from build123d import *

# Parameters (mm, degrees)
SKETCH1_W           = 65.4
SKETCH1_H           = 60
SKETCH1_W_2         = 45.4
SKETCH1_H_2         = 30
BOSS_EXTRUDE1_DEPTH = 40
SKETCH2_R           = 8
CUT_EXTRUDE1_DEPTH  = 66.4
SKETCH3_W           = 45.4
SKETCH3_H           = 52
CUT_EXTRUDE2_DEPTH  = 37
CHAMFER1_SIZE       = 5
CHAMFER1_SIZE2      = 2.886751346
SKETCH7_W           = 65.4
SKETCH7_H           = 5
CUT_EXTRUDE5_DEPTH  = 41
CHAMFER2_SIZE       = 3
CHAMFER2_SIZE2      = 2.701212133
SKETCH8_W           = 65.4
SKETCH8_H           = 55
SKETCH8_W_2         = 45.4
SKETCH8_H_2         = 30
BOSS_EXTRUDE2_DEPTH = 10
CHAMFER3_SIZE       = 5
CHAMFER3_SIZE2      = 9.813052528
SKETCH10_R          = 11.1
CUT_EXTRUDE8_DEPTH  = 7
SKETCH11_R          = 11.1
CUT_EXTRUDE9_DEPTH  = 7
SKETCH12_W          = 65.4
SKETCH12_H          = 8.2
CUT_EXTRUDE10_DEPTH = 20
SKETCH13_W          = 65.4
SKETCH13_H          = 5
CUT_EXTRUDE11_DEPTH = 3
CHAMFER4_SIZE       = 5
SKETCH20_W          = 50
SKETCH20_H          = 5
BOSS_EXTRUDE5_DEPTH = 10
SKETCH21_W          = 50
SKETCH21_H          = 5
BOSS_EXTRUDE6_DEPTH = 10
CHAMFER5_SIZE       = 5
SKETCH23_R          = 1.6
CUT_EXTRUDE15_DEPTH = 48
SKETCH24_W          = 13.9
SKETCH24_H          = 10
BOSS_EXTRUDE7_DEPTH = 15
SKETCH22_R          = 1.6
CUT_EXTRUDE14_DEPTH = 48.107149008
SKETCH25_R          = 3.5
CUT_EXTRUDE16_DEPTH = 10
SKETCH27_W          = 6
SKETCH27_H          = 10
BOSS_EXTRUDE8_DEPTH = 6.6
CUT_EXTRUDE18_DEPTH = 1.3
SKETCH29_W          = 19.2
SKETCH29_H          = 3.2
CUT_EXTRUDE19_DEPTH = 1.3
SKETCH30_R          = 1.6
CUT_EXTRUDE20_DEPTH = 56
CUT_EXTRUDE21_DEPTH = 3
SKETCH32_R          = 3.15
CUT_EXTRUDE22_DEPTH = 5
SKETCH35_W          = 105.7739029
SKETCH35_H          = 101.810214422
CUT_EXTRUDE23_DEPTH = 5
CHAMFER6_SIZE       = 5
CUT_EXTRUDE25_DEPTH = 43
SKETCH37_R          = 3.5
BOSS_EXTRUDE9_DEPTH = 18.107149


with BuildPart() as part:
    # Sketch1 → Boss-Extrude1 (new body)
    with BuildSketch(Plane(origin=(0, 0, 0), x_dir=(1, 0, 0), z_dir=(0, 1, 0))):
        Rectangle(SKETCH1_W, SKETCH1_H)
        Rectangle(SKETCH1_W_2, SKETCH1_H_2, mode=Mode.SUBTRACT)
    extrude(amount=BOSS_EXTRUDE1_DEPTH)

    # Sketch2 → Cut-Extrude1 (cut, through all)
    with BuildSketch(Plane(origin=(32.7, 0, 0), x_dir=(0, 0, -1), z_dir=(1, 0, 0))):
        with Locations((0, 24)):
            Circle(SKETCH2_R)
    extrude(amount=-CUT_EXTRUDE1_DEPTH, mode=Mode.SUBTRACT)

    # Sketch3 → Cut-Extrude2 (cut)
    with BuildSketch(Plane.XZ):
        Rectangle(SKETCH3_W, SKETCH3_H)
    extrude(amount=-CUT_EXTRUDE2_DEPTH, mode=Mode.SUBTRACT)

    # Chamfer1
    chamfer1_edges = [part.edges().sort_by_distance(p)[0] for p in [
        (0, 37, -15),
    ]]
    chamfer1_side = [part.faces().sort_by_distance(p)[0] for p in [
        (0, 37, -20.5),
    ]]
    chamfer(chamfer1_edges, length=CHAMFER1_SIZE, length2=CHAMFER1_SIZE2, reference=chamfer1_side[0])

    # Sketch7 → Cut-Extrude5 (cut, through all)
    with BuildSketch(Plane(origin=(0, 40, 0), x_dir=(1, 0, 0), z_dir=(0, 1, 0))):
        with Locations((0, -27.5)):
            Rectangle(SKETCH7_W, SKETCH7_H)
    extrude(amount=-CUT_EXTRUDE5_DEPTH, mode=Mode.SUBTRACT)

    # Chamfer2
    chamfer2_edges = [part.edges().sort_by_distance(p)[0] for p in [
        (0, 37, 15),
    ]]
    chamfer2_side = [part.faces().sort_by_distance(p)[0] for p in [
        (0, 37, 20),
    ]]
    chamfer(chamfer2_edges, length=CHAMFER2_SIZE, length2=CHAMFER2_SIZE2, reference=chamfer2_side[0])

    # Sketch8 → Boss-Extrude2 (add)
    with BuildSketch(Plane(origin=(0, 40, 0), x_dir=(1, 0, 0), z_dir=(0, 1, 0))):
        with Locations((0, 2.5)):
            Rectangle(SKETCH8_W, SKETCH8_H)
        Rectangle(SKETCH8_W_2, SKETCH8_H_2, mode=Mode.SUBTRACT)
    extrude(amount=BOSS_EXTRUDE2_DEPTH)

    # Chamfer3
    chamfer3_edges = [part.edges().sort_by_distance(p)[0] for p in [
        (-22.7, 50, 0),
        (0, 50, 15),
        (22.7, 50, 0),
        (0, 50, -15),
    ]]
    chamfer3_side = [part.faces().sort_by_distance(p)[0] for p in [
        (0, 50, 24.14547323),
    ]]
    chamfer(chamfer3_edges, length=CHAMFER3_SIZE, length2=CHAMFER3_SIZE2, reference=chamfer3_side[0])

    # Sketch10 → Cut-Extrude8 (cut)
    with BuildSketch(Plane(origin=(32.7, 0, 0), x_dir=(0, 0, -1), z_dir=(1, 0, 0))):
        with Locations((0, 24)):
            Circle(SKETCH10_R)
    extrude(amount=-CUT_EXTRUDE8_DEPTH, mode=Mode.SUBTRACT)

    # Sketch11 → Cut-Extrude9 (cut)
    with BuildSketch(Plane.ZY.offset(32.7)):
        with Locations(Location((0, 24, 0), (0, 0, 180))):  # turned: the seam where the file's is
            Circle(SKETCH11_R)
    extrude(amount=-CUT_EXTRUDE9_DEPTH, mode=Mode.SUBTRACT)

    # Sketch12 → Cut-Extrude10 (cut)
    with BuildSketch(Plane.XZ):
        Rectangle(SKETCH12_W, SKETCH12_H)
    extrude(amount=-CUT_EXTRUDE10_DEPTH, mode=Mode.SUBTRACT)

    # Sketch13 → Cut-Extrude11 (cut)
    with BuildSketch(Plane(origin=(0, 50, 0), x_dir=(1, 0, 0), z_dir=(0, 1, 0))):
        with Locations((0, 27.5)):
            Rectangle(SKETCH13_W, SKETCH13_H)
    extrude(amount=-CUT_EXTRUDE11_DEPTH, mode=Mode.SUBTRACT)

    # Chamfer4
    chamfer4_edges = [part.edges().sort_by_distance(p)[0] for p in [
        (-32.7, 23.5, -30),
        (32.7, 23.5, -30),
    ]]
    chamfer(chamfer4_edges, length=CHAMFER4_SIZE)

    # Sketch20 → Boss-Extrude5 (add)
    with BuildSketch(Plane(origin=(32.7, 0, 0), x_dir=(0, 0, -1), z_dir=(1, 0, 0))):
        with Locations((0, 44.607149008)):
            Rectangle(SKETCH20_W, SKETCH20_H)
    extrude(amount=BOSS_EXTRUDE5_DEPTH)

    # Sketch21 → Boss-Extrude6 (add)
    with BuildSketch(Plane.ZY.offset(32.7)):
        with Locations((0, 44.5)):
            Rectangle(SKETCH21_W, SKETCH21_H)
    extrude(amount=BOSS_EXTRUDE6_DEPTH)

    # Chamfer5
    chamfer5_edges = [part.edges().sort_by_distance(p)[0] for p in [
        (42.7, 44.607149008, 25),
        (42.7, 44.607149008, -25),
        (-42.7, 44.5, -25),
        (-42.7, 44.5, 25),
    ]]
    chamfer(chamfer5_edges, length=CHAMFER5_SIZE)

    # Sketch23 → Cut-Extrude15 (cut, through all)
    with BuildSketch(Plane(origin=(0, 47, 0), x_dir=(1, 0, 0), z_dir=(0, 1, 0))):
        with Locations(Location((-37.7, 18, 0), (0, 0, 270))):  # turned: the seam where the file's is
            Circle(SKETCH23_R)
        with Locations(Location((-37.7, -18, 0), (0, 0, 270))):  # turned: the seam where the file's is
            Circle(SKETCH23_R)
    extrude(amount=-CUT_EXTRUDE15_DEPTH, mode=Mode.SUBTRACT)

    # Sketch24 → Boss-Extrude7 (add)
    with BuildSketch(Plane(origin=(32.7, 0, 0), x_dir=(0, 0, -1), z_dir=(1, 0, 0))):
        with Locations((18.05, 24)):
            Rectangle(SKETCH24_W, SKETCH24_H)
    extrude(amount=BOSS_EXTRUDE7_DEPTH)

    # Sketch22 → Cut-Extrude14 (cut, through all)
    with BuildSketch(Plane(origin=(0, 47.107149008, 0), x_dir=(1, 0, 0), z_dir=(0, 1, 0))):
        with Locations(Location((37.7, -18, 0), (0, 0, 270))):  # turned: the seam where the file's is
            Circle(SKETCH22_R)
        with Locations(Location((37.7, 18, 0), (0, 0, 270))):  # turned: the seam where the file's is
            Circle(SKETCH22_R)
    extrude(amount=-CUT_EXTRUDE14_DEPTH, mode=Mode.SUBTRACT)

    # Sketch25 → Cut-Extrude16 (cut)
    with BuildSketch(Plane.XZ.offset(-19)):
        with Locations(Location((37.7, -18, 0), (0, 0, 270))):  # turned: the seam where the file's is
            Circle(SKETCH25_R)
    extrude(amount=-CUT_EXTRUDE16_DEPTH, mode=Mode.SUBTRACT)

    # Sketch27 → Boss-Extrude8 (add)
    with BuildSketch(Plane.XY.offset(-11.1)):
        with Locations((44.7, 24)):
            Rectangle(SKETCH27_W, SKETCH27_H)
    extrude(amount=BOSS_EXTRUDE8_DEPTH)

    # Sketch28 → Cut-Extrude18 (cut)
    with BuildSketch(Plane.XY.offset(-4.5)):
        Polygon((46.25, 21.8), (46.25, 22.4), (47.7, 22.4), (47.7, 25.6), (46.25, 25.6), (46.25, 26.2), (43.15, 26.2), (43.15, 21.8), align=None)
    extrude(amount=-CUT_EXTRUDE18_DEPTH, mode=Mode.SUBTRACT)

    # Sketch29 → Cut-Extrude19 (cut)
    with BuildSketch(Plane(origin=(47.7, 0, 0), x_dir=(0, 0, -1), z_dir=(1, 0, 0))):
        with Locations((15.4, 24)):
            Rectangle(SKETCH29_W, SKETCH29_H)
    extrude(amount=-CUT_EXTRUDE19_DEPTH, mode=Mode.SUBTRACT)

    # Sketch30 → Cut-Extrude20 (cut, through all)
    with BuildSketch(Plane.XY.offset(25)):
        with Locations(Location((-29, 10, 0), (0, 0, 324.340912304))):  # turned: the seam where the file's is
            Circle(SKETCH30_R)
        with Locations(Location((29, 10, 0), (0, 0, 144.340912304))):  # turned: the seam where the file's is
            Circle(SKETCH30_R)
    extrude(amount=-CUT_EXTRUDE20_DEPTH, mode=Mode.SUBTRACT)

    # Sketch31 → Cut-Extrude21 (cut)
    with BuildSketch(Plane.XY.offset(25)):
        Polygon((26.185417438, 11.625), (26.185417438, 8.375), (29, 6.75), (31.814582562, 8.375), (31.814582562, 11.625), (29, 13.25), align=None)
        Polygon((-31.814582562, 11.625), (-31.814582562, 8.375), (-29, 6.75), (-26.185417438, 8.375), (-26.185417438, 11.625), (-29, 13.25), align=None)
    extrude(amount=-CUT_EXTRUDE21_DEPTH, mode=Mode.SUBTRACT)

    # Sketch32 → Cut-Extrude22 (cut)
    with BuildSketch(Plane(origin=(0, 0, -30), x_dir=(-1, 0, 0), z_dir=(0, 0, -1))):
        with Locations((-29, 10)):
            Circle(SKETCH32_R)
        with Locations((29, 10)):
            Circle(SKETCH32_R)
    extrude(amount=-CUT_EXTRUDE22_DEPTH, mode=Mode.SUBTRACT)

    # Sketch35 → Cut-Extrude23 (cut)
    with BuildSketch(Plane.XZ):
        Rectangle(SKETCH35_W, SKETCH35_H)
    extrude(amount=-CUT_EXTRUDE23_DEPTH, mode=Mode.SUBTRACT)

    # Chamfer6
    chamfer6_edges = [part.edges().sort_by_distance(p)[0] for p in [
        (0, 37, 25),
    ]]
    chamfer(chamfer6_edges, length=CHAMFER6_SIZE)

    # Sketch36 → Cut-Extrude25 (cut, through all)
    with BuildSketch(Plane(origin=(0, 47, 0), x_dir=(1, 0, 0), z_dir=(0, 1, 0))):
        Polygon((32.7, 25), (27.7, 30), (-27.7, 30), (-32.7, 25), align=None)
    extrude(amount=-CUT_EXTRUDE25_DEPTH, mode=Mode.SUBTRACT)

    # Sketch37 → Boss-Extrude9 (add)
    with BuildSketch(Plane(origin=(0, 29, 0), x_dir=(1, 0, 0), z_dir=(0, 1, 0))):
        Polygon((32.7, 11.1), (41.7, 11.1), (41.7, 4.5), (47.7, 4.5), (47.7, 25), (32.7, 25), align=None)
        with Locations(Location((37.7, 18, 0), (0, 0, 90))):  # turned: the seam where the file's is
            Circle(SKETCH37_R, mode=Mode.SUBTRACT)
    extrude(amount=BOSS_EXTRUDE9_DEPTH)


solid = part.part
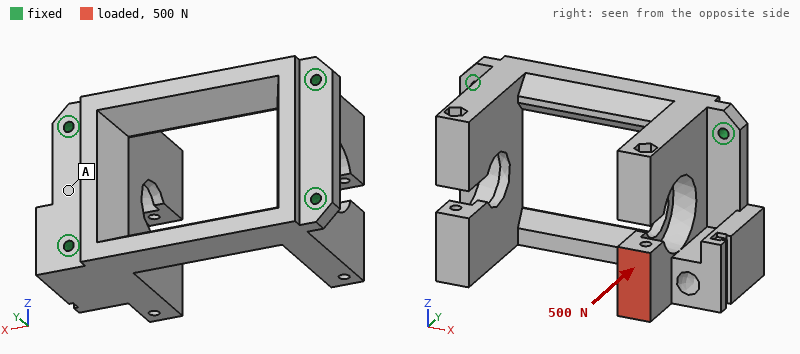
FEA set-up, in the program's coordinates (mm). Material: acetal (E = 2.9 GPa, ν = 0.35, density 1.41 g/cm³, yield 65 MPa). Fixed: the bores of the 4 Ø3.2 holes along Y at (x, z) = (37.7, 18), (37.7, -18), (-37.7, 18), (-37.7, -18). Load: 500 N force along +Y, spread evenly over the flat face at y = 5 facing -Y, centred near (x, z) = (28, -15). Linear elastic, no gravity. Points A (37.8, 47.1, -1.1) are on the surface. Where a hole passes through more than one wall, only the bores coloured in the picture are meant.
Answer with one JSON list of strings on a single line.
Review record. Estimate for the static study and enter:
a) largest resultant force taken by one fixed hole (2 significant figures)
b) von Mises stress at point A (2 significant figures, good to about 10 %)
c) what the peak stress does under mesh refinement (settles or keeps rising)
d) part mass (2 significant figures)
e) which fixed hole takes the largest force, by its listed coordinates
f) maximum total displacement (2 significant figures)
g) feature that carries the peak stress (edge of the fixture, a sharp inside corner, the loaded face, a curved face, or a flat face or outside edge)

["410 N", "1.7 MPa", "keeps rising", "74 g", "(37.7, -18)", "0.38 mm", "edge of the fixture"]
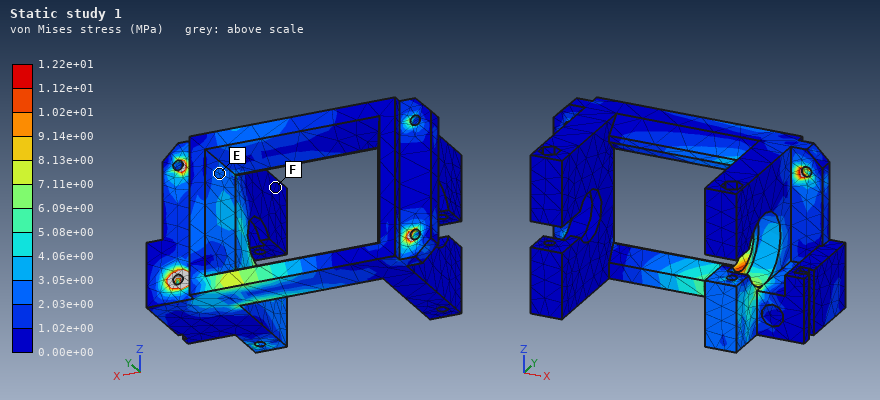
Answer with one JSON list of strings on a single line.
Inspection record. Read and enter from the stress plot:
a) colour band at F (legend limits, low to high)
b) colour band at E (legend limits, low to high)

["0.00e+00 to 1.02e+00 MPa", "2.03e+00 to 3.05e+00 MPa"]
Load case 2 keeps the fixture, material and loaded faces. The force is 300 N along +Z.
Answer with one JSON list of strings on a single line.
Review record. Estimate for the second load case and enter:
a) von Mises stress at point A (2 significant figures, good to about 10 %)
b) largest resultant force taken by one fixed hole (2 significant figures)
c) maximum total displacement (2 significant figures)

["6.8 MPa", "320 N", "0.70 mm"]
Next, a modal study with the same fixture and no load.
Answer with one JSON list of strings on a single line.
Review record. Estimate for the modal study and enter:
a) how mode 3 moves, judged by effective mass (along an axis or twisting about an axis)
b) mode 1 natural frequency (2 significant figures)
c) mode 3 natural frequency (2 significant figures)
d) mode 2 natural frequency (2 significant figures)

["along X", "810 Hz", "1200 Hz", "1100 Hz"]
